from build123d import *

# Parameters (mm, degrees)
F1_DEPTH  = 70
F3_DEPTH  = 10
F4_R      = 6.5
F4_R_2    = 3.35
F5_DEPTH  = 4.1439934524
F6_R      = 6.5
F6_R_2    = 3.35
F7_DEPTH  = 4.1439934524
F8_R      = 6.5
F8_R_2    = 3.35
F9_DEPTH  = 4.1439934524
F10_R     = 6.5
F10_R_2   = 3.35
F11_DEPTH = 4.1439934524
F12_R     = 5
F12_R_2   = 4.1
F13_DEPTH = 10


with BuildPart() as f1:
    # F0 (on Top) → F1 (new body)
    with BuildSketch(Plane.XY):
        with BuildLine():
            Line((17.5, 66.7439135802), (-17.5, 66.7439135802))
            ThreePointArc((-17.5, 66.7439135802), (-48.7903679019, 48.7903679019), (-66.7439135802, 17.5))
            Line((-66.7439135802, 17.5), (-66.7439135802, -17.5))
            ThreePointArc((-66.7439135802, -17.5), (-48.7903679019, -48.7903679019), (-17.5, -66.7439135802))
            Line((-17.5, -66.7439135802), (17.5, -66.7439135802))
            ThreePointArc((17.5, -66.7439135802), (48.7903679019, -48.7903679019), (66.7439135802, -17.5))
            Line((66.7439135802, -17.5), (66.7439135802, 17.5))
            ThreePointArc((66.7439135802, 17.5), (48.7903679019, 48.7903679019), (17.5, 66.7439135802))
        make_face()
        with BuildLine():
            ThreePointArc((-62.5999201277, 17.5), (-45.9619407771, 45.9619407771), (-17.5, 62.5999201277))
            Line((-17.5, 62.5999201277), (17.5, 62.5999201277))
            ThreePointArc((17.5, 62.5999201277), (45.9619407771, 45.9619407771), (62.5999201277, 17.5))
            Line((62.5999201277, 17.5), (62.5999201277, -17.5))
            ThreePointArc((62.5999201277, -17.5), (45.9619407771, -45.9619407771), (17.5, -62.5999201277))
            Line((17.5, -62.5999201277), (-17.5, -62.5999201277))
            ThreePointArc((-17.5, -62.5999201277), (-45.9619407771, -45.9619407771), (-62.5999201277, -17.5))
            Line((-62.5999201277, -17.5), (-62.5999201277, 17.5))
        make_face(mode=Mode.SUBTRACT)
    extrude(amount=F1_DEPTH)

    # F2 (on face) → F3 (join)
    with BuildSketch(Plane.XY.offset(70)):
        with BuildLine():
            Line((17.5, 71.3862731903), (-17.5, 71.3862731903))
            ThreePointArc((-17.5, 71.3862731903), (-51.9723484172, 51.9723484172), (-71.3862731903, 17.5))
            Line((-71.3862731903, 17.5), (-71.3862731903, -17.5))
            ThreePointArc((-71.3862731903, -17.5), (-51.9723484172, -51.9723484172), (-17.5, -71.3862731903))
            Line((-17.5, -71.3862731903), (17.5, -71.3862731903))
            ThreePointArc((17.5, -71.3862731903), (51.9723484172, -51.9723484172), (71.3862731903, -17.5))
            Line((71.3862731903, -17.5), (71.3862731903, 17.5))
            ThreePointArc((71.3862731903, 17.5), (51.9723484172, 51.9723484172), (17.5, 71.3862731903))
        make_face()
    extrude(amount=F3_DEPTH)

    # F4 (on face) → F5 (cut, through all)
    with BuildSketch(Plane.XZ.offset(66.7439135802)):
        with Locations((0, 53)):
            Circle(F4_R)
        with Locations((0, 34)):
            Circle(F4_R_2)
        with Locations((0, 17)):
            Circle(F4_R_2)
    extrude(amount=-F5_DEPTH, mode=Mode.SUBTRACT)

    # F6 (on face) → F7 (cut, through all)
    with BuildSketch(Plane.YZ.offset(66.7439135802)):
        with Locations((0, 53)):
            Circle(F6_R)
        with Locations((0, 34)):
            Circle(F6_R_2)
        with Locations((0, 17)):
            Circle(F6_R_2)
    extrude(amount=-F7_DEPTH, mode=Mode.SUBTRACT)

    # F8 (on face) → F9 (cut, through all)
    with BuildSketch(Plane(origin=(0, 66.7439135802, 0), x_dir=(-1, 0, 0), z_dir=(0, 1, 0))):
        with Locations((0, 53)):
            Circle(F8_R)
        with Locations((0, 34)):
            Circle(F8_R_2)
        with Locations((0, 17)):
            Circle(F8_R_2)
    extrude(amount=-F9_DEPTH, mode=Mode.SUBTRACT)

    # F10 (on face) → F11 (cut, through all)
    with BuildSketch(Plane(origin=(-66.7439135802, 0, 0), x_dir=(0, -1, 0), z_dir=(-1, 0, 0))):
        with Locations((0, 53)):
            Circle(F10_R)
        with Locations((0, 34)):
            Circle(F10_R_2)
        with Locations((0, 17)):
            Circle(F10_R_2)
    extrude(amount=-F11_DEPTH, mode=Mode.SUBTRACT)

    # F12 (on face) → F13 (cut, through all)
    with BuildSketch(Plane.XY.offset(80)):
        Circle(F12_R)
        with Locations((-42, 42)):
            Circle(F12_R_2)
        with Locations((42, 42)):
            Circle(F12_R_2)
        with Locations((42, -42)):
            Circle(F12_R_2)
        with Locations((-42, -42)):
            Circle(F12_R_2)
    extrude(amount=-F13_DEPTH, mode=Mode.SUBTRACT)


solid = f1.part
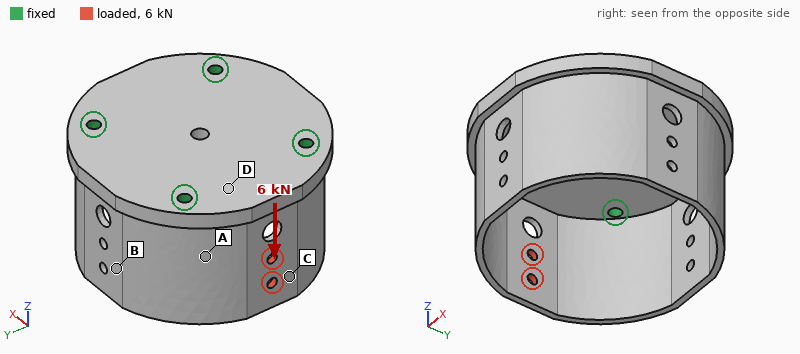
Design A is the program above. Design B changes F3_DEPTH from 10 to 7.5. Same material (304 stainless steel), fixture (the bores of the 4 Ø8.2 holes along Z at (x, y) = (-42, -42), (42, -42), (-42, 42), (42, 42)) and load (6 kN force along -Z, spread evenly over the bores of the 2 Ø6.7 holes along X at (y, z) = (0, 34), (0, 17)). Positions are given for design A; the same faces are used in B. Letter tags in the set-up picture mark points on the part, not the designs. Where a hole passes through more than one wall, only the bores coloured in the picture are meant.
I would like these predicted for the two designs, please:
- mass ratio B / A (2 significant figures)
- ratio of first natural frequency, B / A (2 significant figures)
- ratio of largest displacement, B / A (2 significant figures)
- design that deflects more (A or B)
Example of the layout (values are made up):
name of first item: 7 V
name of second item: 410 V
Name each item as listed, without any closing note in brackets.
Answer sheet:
mass ratio B / A: 0.85
ratio of first natural frequency, B / A: 0.83
ratio of largest displacement, B / A: 1.4
design that deflects more: B
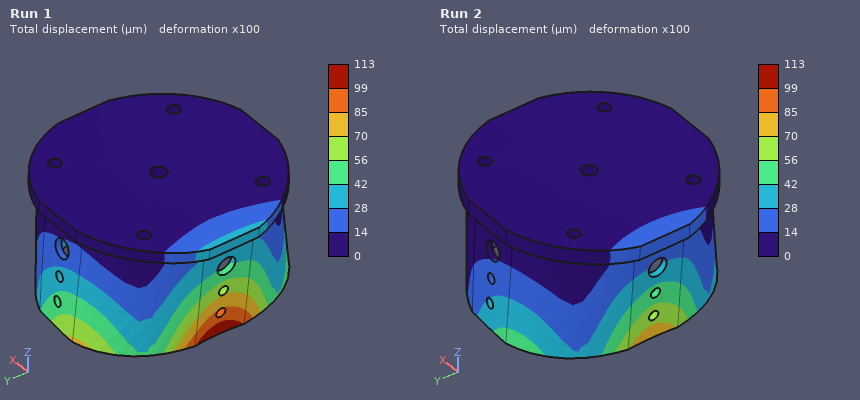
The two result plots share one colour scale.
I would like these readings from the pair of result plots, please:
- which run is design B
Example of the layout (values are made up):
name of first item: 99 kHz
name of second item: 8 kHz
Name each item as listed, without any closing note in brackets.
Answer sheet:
which run is design B: Run 1
